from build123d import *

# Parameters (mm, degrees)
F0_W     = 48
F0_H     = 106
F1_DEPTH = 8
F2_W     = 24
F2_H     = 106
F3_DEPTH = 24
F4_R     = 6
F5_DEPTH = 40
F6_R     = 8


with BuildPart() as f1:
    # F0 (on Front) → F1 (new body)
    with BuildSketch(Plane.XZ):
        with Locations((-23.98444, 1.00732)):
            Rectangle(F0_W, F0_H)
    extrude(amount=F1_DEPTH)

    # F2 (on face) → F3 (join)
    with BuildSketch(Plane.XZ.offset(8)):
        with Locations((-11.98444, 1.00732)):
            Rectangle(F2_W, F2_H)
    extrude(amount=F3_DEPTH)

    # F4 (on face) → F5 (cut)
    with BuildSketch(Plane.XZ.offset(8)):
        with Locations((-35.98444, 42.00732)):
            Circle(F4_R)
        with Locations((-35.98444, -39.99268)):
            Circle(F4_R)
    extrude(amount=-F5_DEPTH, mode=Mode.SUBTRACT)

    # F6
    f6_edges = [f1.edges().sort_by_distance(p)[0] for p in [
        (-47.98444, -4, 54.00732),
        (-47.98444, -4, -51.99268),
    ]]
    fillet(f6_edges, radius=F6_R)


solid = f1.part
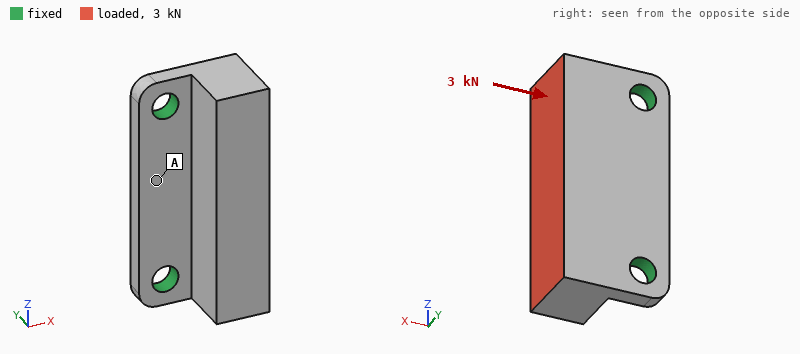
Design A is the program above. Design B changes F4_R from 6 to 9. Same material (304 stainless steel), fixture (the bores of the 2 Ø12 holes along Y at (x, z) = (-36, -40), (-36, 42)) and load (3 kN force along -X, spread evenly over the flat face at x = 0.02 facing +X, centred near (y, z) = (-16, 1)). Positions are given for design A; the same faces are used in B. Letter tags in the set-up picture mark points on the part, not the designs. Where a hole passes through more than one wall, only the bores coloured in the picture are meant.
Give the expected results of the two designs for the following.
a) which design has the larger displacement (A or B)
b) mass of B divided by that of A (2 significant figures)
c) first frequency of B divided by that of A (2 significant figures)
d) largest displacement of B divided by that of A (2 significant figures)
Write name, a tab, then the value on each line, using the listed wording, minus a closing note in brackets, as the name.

which design has the larger displacement	A
mass of B divided by that of A	0.98
first frequency of B divided by that of A	1.2
largest displacement of B divided by that of A	0.70
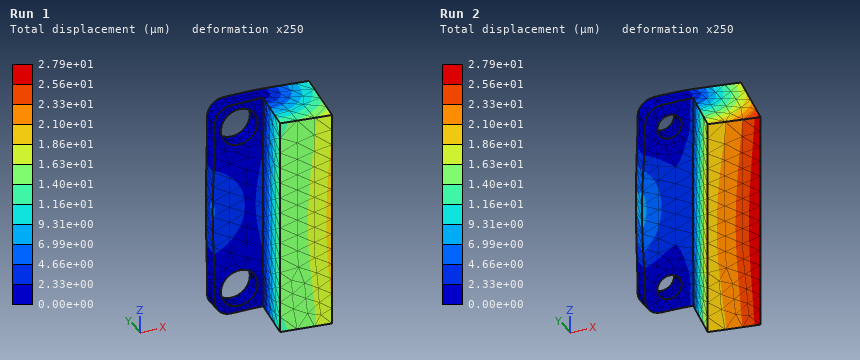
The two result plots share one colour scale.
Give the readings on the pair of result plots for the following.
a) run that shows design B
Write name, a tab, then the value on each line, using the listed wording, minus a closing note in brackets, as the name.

run that shows design B	Run 1
